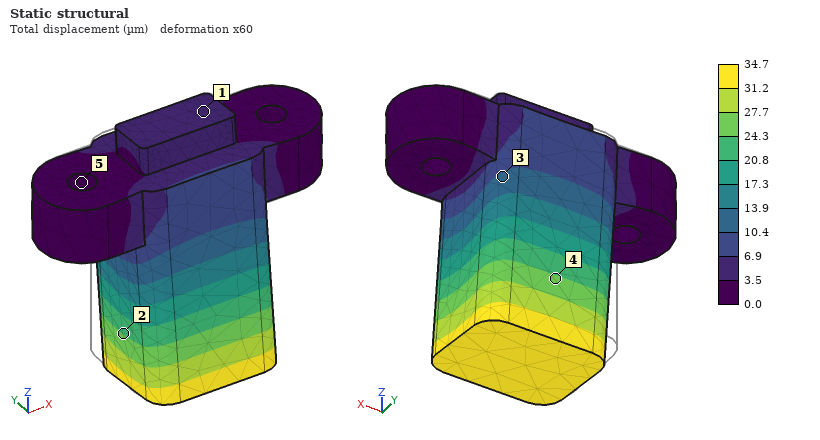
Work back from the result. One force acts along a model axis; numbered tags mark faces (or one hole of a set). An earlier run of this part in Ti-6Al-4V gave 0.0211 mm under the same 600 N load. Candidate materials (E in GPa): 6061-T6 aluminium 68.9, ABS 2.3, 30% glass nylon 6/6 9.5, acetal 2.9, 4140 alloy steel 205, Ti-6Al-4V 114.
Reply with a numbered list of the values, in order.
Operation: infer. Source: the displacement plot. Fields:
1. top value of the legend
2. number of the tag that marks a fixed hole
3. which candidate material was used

1. 34.7 µm
2. 5
3. 6061-T6 aluminium
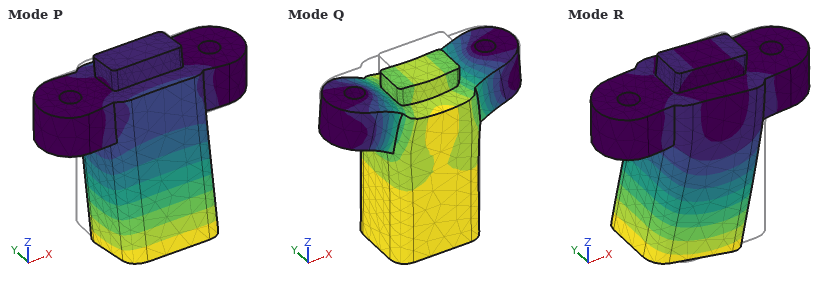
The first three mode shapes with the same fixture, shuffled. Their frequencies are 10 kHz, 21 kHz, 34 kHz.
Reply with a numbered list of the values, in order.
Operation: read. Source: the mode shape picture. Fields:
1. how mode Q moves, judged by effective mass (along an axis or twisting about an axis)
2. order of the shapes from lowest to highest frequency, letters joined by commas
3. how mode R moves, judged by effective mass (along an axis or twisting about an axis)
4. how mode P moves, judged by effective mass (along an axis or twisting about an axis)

1. along Z
2. P, R, Q
3. along X
4. along Y
